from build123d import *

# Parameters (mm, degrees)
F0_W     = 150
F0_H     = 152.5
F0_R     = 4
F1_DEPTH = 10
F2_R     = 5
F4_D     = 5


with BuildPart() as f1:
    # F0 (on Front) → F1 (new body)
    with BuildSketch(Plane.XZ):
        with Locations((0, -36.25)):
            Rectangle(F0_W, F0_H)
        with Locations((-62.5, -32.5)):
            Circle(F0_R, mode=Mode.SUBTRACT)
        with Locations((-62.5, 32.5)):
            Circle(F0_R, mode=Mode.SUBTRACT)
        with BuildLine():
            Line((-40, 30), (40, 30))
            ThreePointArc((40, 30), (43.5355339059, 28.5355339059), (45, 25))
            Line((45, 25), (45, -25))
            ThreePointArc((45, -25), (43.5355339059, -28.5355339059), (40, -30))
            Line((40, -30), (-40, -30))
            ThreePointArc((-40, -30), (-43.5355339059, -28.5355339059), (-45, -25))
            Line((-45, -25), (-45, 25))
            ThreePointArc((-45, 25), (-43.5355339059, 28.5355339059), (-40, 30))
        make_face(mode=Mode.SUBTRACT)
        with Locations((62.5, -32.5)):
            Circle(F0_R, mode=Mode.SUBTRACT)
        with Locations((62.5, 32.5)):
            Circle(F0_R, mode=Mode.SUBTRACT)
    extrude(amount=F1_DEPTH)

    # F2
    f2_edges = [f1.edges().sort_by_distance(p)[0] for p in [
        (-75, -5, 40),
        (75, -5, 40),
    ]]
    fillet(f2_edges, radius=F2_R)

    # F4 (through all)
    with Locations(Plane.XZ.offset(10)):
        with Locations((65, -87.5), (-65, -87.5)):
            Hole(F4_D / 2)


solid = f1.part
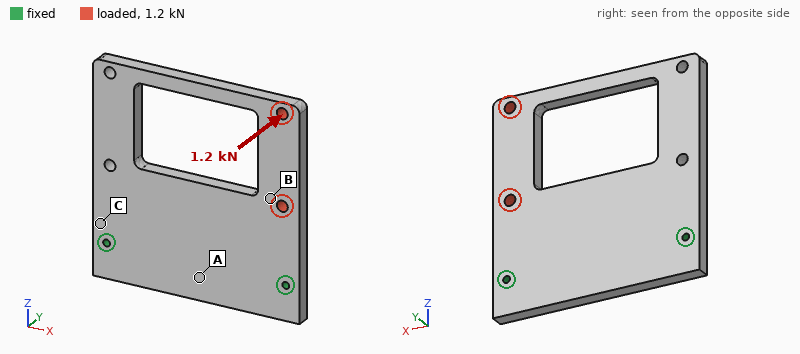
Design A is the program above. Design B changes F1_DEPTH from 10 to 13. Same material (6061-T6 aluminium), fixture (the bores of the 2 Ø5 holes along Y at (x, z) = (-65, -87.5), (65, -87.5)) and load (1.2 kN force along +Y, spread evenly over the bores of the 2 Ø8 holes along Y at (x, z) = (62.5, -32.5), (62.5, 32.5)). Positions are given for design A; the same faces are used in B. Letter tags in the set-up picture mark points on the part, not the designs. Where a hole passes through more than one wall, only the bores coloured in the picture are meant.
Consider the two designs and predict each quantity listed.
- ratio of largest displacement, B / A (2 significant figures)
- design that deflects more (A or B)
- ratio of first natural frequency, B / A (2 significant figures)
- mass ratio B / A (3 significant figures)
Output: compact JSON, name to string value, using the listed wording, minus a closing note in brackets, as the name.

{"ratio of largest displacement, B / A": "0.48", "design that deflects more": "A", "ratio of first natural frequency, B / A": "1.3", "mass ratio B / A": "1.30"}
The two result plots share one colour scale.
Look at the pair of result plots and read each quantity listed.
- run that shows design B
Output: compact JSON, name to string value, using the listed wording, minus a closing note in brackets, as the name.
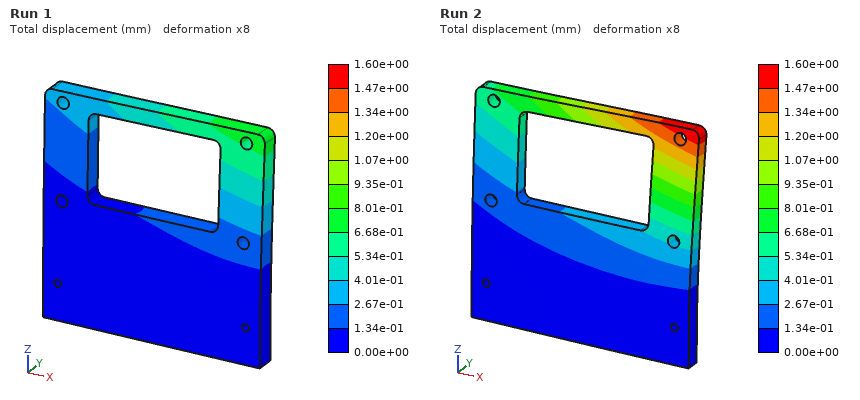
{"run that shows design B": "Run 1"}
